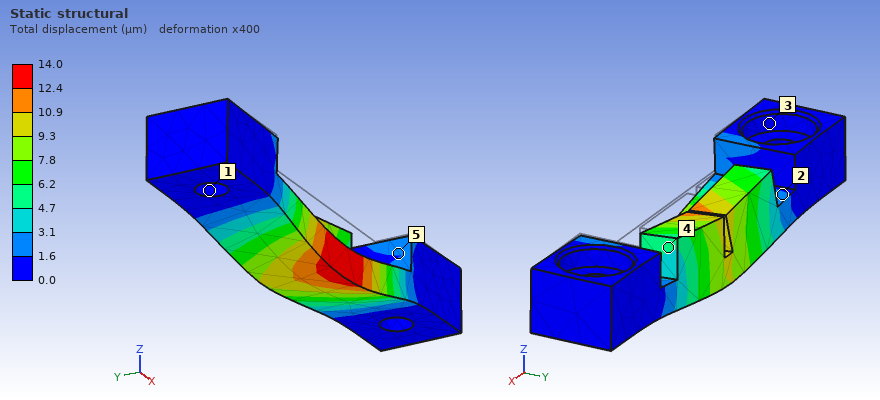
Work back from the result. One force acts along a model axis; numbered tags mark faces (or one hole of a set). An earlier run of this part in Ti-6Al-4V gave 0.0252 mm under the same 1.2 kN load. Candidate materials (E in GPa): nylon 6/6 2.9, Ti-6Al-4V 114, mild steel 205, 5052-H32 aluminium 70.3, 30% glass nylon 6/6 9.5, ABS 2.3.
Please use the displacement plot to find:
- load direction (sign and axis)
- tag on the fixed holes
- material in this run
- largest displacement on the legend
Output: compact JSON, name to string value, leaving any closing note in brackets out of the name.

{"load direction": "-Z", "tag on the fixed holes": "1", "material in this run": "mild steel", "largest displacement on the legend": "14.0 µm"}
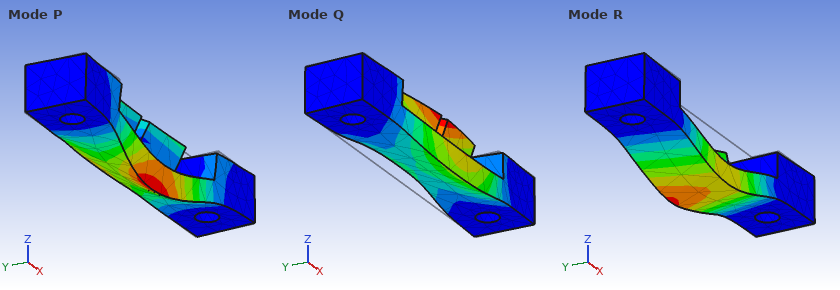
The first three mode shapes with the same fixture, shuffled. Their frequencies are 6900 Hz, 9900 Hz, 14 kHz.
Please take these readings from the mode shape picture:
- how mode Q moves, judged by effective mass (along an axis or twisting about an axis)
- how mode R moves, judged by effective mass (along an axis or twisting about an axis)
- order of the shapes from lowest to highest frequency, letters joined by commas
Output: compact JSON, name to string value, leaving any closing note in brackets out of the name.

{"how mode Q moves, judged by effective mass": "along Y", "how mode R moves, judged by effective mass": "along Z", "order of the shapes from lowest to highest frequency, letters joined by commas": "R, Q, P"}
